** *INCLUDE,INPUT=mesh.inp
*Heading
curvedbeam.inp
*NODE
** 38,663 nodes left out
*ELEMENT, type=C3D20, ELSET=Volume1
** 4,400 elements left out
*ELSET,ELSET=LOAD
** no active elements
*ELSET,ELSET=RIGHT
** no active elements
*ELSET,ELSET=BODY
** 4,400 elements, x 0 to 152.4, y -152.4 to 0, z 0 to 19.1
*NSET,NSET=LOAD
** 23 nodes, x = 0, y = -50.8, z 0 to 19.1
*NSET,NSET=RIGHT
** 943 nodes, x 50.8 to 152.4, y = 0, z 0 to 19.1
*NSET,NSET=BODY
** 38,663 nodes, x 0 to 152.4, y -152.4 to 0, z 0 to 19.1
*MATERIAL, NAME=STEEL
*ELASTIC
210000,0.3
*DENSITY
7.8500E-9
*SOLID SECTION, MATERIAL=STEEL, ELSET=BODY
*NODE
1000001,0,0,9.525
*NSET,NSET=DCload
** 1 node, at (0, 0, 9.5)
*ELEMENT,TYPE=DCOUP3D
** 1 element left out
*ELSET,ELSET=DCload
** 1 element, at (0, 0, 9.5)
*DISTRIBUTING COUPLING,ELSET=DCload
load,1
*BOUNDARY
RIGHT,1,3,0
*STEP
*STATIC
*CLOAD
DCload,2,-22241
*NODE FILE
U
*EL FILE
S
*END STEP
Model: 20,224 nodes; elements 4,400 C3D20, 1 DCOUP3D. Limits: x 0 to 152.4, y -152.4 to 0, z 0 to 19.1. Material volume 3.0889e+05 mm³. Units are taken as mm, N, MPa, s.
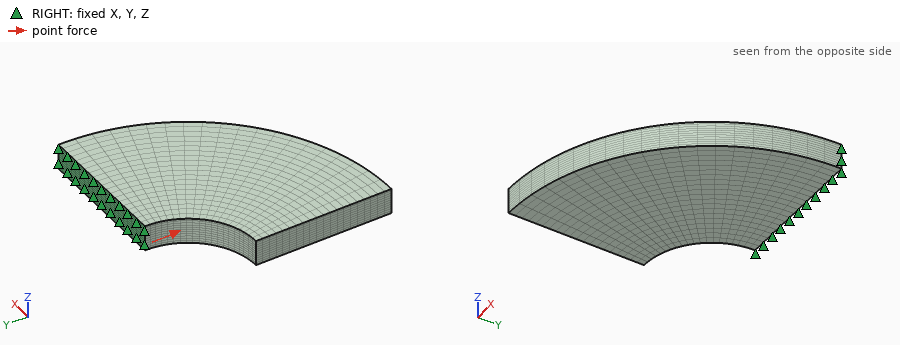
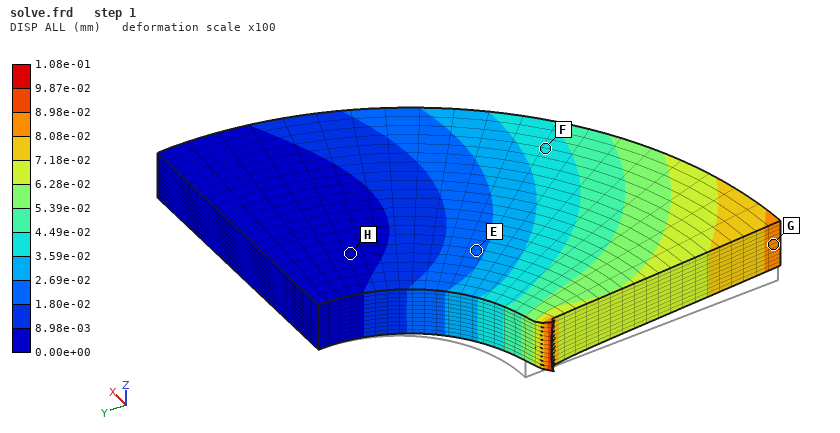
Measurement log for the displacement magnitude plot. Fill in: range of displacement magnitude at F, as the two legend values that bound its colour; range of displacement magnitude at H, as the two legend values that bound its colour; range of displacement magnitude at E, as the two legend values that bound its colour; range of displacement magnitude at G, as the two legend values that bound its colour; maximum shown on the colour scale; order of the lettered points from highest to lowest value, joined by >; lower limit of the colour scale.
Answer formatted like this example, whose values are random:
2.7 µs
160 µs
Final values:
3.59e-02 to 4.49e-02 mm
0.00e+00 to 8.98e-03 mm
1.80e-02 to 2.69e-02 mm
8.08e-02 to 8.98e-02 mm
1.08e-01 mm
G > F > E > H
0.00e+00 mm
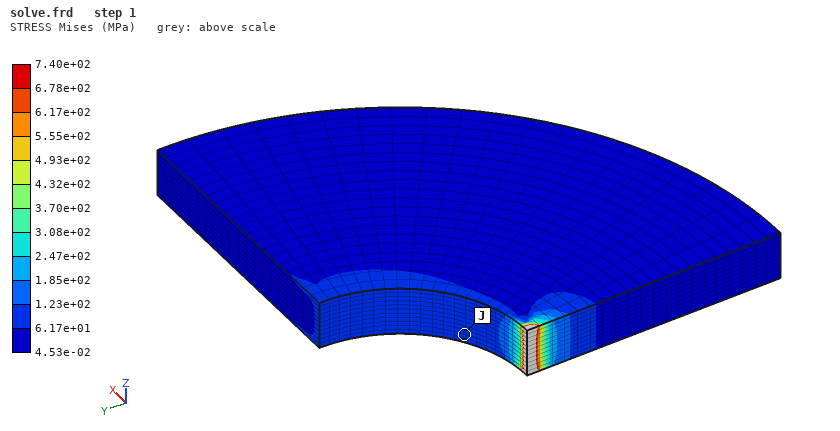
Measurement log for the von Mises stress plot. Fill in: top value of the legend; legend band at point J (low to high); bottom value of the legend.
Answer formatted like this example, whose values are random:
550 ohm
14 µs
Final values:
7.40e+02 MPa
6.17e+01 to 1.23e+02 MPa
4.53e-02 MPa
